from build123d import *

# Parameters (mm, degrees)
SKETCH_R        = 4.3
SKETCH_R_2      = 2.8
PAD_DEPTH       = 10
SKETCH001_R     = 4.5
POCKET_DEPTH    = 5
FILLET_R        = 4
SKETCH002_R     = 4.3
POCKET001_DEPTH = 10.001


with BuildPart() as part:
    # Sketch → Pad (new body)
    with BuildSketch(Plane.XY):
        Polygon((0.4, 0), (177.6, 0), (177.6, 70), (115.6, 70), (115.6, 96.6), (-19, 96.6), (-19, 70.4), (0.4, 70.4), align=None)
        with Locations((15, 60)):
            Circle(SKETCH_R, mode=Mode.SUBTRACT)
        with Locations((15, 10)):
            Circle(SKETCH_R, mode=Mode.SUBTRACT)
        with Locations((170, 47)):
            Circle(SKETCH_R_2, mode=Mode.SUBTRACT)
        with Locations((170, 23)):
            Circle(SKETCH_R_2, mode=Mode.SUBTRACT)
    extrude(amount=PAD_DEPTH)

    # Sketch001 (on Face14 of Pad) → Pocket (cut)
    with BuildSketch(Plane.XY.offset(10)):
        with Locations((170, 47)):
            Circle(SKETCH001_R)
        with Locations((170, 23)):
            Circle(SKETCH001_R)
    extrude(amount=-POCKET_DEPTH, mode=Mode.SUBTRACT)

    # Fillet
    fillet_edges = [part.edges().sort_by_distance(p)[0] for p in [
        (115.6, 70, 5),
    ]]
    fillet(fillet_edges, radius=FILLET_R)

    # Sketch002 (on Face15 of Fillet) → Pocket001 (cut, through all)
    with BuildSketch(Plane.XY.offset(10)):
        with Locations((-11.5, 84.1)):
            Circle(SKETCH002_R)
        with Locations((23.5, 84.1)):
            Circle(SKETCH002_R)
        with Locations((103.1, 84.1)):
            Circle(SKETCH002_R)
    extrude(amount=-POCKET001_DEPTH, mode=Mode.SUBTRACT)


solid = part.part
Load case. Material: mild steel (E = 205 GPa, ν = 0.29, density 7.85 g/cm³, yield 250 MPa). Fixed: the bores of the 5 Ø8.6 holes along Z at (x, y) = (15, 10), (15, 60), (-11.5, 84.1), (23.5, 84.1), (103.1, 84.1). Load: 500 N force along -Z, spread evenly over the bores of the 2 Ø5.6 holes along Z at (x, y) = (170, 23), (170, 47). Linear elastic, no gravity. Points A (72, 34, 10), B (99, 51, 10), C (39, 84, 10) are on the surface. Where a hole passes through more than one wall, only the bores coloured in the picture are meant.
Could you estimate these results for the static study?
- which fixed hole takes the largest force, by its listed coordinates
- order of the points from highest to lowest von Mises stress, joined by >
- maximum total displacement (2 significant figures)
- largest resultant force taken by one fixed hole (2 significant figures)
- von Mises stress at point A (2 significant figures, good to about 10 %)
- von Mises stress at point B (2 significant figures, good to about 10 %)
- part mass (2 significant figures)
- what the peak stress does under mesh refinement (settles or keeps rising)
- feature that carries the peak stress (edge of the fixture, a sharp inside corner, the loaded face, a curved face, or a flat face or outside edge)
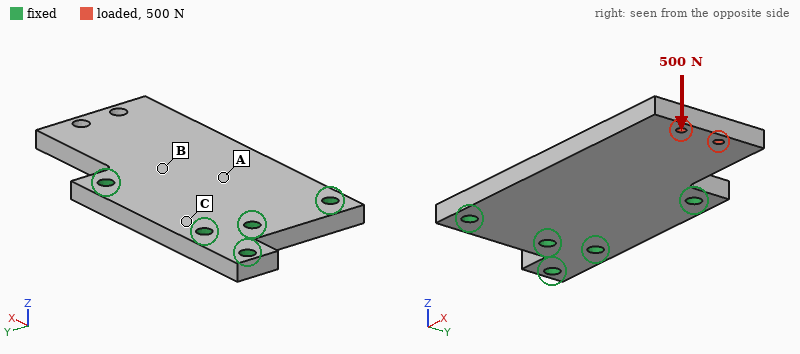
(103.1, 84.1)
B > A > C
0.14 mm
760 N
14 MPa
24 MPa
1.2 kg
keeps rising
edge of the fixture
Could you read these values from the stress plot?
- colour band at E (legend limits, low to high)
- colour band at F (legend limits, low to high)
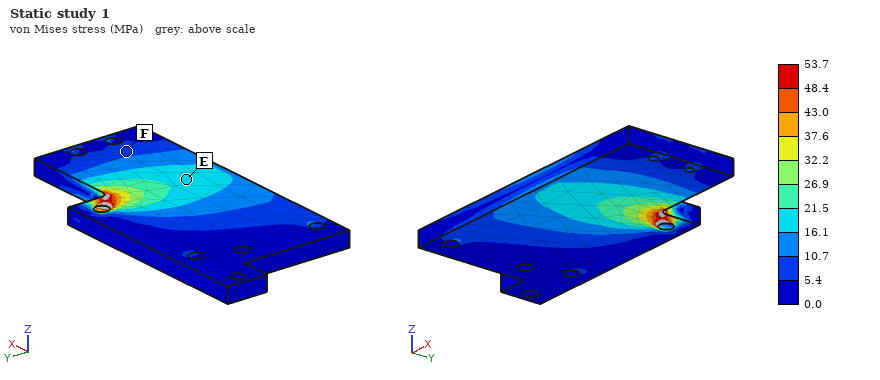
16.1 to 21.5 MPa
5.4 to 10.7 MPa
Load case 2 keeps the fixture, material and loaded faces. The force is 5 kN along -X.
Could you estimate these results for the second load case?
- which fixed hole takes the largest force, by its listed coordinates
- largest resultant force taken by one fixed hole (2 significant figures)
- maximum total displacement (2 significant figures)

(15, 10)
1.9 kN
48 µm
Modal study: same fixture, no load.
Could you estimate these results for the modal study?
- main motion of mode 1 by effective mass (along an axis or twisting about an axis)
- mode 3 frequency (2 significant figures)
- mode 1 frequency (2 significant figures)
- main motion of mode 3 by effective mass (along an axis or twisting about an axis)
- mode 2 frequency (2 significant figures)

along Z
3600 Hz
790 Hz
along Z
2000 Hz
